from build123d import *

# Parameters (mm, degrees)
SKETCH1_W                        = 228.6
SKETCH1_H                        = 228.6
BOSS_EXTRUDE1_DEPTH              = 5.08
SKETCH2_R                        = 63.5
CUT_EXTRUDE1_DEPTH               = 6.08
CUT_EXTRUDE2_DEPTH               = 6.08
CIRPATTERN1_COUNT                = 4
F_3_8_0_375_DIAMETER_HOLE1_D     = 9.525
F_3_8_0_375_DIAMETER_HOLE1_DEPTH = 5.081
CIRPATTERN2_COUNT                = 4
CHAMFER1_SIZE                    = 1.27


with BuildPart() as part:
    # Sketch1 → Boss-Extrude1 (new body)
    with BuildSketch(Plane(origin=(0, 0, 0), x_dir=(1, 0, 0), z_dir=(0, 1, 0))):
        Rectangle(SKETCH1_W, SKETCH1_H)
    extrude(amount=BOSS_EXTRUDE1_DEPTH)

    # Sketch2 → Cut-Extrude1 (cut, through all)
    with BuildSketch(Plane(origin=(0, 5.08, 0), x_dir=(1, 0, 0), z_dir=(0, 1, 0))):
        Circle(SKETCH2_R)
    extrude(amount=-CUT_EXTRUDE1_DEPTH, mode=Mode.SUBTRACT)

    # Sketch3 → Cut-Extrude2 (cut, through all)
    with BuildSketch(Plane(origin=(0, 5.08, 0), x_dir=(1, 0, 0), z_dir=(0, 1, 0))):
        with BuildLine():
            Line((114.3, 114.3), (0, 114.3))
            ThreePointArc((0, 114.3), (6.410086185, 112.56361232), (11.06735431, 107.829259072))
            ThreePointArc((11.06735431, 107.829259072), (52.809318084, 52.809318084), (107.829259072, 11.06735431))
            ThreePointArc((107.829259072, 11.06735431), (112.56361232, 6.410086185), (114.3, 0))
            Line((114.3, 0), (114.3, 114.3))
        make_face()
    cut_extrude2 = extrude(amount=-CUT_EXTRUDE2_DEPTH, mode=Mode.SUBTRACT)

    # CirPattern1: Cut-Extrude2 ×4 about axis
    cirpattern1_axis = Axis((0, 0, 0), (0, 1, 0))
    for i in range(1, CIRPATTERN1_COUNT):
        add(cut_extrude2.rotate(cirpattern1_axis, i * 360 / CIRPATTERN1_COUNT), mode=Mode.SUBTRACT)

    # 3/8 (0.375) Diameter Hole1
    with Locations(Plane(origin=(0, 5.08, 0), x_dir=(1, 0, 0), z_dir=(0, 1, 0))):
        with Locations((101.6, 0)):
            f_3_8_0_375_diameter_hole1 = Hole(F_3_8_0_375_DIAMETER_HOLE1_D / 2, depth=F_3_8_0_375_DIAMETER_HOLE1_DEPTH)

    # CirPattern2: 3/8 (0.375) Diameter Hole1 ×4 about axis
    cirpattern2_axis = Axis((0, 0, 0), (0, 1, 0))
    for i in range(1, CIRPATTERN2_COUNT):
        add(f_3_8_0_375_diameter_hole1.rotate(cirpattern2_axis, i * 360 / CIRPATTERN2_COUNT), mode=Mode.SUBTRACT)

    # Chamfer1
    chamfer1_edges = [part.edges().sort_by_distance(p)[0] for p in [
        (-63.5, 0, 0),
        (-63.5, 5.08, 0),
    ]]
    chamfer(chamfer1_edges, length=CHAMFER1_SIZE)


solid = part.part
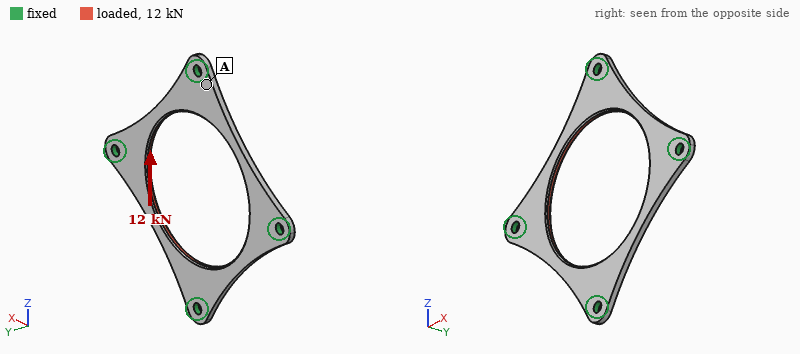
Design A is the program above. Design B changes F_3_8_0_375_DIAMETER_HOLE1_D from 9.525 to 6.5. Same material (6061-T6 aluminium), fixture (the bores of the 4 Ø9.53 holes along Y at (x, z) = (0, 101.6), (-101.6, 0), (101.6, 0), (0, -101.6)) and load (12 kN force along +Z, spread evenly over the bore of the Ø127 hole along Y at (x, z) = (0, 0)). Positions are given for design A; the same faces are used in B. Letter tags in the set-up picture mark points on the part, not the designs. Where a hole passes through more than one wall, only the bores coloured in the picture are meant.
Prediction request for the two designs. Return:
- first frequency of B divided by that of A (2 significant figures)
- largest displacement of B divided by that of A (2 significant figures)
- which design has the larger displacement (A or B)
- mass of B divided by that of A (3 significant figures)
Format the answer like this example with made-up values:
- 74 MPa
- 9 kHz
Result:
- 0.92
- 1.2
- B
- 1.01
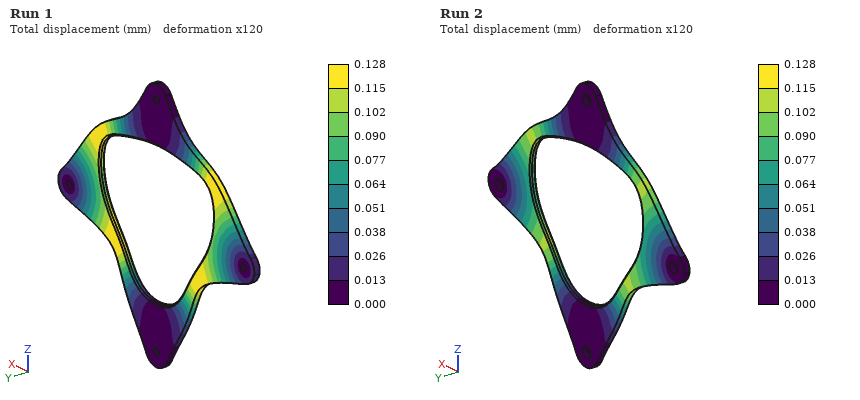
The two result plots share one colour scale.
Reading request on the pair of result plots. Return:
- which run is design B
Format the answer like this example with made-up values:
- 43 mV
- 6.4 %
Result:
- Run 1
